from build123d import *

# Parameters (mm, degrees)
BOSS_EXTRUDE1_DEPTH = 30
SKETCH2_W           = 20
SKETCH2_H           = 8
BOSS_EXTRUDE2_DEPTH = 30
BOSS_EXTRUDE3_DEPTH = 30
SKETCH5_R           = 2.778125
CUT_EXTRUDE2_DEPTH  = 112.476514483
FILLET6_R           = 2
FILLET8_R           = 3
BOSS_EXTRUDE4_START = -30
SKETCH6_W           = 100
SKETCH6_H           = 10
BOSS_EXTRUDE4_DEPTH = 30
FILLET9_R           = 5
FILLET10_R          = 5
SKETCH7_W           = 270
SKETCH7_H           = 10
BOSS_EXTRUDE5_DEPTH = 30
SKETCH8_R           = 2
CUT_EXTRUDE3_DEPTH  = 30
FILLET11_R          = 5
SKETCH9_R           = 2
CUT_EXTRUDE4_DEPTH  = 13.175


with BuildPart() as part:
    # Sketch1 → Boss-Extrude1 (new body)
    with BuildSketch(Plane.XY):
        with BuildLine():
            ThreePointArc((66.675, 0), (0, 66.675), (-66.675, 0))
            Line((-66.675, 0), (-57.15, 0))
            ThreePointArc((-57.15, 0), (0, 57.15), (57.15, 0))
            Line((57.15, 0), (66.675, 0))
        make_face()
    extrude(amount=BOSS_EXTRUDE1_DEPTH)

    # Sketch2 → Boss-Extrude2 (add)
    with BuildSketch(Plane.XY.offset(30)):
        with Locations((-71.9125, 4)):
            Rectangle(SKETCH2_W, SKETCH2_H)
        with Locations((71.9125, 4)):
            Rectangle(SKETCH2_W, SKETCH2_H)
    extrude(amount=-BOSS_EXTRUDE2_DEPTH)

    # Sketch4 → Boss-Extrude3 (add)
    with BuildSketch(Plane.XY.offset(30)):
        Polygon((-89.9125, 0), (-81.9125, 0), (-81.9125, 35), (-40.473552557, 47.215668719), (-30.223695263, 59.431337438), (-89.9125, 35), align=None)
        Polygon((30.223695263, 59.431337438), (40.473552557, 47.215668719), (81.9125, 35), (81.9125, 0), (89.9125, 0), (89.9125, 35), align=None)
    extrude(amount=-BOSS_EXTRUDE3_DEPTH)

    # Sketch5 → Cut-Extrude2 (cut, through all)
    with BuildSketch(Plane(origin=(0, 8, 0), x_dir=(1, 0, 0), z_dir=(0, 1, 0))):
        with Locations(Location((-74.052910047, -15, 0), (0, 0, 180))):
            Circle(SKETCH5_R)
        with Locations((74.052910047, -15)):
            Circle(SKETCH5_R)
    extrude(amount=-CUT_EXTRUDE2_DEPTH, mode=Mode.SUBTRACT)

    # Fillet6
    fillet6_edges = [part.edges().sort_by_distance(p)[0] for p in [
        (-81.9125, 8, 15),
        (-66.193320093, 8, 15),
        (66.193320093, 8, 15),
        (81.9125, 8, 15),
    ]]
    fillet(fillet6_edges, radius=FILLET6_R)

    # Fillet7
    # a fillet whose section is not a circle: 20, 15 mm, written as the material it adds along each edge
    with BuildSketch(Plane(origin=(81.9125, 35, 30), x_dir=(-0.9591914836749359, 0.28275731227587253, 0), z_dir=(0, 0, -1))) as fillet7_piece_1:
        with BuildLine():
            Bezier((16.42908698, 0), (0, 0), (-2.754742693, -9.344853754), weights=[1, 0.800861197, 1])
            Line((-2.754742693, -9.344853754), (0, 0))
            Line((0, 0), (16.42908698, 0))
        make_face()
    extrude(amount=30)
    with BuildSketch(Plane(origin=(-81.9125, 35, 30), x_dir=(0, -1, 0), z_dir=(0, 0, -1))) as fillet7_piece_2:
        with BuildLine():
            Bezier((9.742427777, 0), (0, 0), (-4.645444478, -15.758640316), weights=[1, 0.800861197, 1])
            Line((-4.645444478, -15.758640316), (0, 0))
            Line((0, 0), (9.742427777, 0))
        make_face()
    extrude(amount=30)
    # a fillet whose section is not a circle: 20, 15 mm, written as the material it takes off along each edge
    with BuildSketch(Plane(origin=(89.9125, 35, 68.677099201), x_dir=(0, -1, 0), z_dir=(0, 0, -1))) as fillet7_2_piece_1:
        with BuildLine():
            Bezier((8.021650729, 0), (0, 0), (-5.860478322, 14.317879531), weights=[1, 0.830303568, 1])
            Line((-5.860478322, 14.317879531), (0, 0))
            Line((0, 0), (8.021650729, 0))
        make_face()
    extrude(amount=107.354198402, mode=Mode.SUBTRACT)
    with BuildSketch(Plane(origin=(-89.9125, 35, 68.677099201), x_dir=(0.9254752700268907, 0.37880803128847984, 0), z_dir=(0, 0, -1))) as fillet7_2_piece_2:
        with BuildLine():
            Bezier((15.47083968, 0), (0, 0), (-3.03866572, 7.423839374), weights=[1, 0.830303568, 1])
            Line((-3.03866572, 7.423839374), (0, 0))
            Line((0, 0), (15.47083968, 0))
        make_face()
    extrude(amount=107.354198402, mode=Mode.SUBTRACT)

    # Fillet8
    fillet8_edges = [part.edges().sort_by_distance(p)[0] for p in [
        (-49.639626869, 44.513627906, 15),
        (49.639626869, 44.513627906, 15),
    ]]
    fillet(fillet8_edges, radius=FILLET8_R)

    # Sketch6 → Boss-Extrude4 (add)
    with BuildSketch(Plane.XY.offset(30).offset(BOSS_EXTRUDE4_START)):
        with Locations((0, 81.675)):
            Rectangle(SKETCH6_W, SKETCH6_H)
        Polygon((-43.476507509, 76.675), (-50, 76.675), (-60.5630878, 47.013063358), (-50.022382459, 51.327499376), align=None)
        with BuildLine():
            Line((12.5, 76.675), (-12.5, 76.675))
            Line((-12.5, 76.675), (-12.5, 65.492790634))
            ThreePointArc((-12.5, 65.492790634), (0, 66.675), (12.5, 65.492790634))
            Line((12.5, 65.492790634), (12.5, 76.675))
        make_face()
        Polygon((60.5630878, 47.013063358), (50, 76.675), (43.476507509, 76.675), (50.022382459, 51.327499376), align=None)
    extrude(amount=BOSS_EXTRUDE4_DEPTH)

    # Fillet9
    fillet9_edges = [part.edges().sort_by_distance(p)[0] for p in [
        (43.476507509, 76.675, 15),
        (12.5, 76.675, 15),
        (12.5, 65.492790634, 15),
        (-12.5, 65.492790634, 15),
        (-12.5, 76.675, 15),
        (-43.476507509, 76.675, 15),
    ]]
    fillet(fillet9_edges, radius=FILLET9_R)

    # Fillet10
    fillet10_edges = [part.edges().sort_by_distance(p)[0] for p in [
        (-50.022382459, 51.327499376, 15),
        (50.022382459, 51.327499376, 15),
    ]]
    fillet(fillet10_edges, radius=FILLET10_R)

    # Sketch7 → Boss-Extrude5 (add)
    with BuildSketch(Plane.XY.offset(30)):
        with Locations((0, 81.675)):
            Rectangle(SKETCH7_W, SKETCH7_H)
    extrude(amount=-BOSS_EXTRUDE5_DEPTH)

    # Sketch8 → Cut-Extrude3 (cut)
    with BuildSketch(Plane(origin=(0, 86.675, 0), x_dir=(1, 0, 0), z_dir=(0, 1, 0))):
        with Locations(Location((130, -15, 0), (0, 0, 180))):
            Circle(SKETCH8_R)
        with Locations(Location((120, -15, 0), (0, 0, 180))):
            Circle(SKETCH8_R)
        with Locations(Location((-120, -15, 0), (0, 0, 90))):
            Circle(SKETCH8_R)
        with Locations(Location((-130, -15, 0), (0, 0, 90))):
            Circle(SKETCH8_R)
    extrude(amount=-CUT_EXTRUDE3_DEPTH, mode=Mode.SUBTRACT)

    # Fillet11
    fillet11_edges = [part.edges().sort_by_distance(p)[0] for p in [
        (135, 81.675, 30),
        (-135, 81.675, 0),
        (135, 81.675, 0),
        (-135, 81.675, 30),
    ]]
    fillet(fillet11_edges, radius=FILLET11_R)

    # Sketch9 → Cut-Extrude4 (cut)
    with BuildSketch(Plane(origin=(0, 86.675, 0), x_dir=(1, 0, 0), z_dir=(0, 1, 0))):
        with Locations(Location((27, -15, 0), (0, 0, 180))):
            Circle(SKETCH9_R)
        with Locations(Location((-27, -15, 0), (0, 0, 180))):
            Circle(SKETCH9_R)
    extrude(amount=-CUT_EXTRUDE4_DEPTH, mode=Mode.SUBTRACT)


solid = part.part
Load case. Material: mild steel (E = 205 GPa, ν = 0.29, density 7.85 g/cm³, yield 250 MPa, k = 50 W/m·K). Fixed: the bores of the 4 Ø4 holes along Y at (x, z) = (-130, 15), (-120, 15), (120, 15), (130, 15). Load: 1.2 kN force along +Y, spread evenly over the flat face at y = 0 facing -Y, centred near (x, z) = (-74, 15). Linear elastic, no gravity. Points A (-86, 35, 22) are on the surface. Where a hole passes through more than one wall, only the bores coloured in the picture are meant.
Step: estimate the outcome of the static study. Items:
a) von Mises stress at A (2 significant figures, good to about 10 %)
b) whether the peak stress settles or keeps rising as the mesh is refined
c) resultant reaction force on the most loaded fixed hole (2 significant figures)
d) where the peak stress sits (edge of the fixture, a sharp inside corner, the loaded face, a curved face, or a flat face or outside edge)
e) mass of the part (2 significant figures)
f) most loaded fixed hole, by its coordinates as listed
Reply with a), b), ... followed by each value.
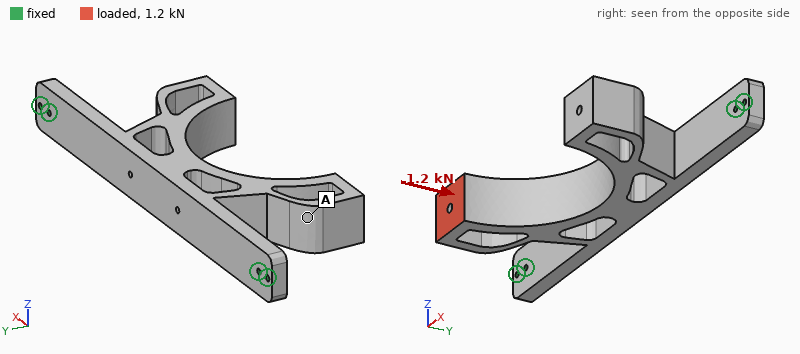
a) 10 MPa
b) keeps rising
c) 2.2 kN
d) edge of the fixture
e) 1.5 kg
f) (-120, 15)
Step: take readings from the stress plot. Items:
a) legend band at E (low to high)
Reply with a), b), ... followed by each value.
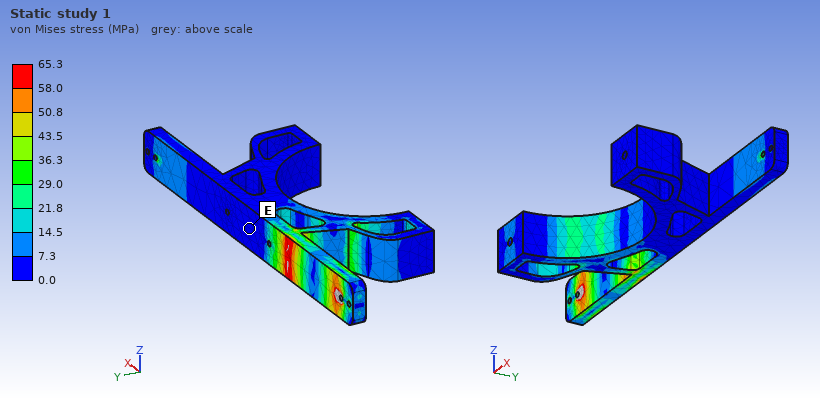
a) 0.0 to 7.3 MPa
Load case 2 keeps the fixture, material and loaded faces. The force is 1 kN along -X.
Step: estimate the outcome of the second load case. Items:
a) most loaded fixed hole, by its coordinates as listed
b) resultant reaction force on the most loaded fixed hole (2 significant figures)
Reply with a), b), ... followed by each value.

a) (120, 15)
b) 1.1 kN
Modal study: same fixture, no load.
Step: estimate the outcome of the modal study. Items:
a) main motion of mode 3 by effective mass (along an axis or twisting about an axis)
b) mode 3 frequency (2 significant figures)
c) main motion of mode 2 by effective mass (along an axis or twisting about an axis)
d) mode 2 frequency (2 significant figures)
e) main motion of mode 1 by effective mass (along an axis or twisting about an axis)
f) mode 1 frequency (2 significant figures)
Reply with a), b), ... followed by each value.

a) along X
b) 810 Hz
c) along Y
d) 640 Hz
e) along Z
f) 430 Hz
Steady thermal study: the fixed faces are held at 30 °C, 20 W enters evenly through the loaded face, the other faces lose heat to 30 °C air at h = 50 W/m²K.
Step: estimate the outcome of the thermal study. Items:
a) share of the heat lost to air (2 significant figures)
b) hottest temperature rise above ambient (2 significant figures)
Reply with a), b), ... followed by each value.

a) 93 %
b) 42 K
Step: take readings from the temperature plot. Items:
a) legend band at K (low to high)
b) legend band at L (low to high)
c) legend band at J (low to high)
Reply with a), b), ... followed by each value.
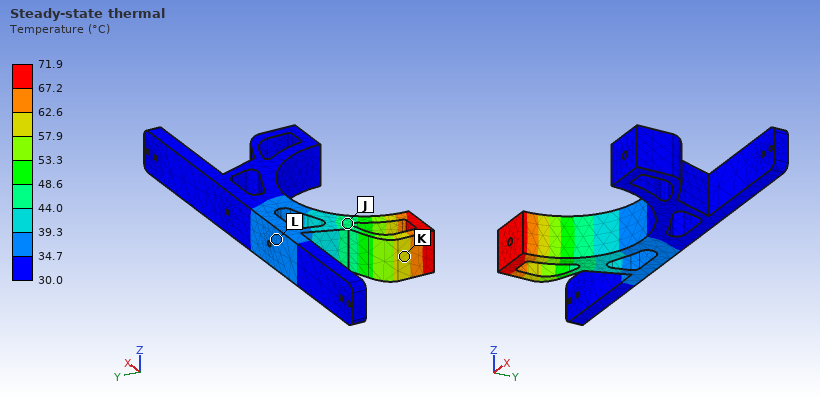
a) 57.9 to 62.6 °C
b) 34.7 to 39.3 °C
c) 44.0 to 48.6 °C
